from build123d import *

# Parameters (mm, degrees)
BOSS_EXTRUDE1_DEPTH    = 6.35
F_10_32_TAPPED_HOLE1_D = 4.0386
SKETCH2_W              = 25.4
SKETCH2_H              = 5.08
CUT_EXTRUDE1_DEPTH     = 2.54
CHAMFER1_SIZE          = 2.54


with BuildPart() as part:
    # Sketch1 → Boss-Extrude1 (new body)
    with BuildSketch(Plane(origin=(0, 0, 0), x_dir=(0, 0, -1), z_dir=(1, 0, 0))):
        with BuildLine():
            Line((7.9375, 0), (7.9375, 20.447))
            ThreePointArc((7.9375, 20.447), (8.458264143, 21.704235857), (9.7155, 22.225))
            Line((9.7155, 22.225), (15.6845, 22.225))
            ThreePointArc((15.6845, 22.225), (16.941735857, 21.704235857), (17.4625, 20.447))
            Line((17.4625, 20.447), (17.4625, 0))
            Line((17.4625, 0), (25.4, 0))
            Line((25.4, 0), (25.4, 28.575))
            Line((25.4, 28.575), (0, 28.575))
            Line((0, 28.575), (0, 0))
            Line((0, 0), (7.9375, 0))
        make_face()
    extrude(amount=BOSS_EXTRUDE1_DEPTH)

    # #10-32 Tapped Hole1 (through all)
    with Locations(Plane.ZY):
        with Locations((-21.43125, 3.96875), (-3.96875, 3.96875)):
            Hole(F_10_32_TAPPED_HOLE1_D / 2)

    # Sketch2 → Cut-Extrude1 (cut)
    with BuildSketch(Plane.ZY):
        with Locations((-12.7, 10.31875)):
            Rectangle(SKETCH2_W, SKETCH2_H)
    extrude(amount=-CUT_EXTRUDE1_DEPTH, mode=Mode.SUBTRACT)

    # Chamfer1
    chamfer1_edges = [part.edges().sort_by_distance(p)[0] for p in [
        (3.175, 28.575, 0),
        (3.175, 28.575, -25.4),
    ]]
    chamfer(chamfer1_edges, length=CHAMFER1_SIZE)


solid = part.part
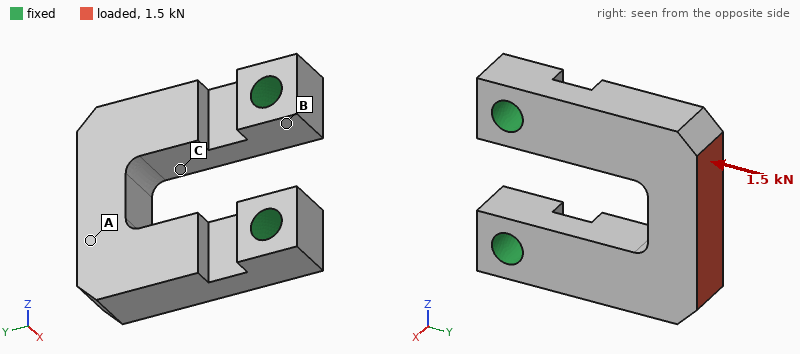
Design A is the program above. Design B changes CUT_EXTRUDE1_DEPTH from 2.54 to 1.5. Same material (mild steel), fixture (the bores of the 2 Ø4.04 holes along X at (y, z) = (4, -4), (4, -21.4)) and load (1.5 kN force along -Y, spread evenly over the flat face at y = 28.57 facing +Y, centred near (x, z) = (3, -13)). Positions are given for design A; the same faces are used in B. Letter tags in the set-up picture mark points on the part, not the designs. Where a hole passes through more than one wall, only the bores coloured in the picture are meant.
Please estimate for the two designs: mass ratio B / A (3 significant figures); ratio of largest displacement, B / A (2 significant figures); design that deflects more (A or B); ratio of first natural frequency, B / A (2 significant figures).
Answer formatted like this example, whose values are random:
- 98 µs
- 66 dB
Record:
- 1.03
- 0.34
- A
- 1.4
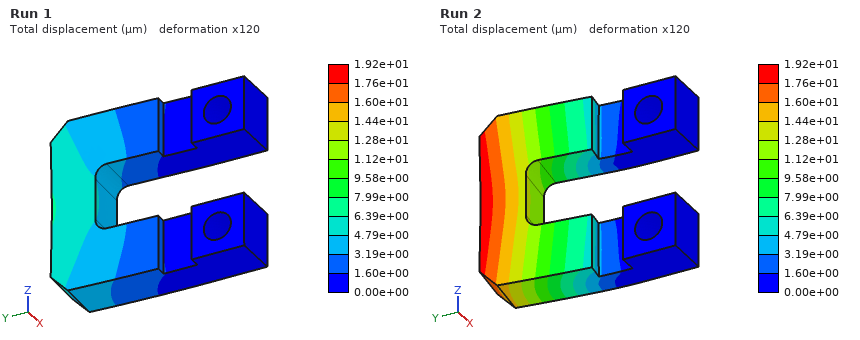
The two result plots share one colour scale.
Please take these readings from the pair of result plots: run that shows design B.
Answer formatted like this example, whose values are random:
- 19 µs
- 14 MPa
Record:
- Run 1
